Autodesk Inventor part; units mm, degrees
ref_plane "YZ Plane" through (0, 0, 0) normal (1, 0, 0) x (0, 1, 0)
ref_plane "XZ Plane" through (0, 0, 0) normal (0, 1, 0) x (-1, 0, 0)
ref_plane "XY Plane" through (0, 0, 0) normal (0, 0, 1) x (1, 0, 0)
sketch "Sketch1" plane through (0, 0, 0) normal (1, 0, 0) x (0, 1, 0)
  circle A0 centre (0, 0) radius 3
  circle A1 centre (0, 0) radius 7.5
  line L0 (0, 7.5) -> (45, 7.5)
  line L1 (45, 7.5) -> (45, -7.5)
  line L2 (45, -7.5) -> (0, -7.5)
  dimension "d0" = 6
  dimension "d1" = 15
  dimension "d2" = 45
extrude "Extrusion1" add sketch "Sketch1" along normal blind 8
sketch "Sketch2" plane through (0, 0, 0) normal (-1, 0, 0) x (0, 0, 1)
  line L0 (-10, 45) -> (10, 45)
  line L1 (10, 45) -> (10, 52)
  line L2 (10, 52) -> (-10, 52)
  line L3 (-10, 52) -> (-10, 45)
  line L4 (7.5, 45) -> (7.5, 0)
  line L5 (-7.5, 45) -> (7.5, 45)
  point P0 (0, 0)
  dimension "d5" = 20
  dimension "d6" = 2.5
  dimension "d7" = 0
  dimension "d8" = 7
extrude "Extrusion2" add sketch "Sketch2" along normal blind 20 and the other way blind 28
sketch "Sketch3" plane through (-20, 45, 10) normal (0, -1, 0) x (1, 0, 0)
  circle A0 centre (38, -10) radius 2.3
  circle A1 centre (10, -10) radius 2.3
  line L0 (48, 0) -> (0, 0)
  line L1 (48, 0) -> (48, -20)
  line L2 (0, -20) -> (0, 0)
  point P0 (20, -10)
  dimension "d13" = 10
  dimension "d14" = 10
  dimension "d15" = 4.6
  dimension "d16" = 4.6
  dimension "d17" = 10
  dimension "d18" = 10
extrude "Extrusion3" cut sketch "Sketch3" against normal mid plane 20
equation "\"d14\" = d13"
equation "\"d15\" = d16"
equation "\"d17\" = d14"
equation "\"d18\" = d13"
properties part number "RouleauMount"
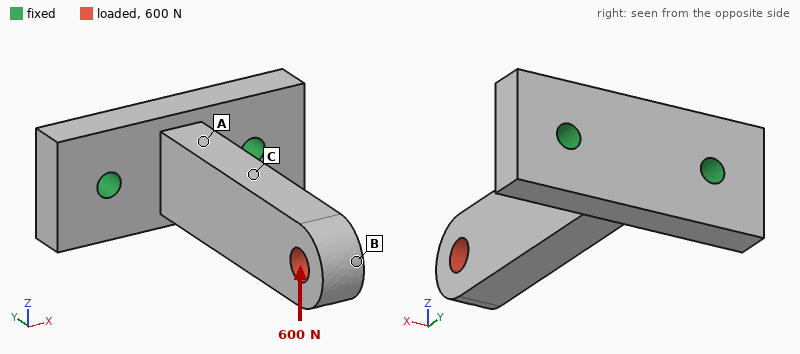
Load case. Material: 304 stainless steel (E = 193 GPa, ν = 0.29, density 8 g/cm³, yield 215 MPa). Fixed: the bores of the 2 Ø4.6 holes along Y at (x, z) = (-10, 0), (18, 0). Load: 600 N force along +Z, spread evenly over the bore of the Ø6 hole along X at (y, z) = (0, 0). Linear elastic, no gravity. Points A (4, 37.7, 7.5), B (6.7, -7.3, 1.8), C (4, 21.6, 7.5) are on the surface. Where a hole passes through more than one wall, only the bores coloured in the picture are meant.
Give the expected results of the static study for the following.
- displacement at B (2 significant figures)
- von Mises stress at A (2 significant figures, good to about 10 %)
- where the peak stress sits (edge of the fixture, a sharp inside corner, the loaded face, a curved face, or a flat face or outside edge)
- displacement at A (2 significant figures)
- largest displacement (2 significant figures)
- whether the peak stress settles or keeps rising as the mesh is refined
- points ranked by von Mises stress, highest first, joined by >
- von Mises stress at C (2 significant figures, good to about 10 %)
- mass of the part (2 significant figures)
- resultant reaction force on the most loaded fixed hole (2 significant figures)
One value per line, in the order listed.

0.12 mm
76 MPa
edge of the fixture
0.019 mm
0.12 mm
keeps rising
A > C > B
43 MPa
99 g
300 N
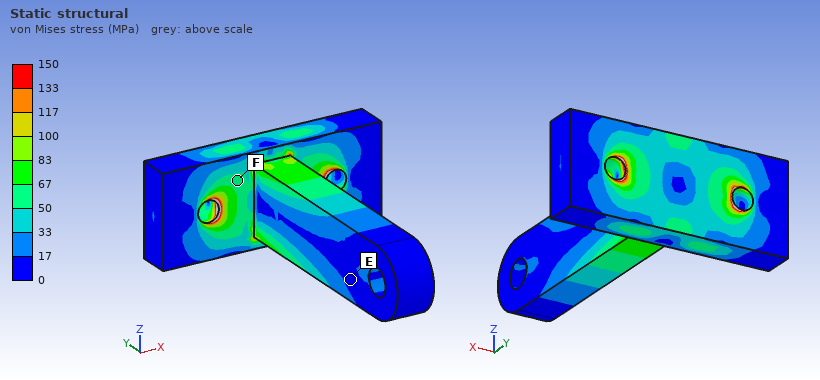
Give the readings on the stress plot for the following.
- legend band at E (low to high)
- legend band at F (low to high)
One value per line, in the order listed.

0 to 17 MPa
50 to 67 MPa
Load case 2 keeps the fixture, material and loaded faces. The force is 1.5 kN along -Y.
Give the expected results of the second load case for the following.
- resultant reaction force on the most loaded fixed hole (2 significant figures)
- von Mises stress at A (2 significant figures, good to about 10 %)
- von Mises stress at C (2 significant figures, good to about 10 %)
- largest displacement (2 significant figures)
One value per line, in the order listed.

760 N
13 MPa
13 MPa
5.8 µm
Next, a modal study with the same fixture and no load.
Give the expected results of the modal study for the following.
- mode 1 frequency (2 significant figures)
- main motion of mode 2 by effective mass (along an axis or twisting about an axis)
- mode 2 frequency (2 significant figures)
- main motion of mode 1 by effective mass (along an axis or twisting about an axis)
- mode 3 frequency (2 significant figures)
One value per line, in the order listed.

2200 Hz
along Z
2900 Hz
along X
12 kHz
